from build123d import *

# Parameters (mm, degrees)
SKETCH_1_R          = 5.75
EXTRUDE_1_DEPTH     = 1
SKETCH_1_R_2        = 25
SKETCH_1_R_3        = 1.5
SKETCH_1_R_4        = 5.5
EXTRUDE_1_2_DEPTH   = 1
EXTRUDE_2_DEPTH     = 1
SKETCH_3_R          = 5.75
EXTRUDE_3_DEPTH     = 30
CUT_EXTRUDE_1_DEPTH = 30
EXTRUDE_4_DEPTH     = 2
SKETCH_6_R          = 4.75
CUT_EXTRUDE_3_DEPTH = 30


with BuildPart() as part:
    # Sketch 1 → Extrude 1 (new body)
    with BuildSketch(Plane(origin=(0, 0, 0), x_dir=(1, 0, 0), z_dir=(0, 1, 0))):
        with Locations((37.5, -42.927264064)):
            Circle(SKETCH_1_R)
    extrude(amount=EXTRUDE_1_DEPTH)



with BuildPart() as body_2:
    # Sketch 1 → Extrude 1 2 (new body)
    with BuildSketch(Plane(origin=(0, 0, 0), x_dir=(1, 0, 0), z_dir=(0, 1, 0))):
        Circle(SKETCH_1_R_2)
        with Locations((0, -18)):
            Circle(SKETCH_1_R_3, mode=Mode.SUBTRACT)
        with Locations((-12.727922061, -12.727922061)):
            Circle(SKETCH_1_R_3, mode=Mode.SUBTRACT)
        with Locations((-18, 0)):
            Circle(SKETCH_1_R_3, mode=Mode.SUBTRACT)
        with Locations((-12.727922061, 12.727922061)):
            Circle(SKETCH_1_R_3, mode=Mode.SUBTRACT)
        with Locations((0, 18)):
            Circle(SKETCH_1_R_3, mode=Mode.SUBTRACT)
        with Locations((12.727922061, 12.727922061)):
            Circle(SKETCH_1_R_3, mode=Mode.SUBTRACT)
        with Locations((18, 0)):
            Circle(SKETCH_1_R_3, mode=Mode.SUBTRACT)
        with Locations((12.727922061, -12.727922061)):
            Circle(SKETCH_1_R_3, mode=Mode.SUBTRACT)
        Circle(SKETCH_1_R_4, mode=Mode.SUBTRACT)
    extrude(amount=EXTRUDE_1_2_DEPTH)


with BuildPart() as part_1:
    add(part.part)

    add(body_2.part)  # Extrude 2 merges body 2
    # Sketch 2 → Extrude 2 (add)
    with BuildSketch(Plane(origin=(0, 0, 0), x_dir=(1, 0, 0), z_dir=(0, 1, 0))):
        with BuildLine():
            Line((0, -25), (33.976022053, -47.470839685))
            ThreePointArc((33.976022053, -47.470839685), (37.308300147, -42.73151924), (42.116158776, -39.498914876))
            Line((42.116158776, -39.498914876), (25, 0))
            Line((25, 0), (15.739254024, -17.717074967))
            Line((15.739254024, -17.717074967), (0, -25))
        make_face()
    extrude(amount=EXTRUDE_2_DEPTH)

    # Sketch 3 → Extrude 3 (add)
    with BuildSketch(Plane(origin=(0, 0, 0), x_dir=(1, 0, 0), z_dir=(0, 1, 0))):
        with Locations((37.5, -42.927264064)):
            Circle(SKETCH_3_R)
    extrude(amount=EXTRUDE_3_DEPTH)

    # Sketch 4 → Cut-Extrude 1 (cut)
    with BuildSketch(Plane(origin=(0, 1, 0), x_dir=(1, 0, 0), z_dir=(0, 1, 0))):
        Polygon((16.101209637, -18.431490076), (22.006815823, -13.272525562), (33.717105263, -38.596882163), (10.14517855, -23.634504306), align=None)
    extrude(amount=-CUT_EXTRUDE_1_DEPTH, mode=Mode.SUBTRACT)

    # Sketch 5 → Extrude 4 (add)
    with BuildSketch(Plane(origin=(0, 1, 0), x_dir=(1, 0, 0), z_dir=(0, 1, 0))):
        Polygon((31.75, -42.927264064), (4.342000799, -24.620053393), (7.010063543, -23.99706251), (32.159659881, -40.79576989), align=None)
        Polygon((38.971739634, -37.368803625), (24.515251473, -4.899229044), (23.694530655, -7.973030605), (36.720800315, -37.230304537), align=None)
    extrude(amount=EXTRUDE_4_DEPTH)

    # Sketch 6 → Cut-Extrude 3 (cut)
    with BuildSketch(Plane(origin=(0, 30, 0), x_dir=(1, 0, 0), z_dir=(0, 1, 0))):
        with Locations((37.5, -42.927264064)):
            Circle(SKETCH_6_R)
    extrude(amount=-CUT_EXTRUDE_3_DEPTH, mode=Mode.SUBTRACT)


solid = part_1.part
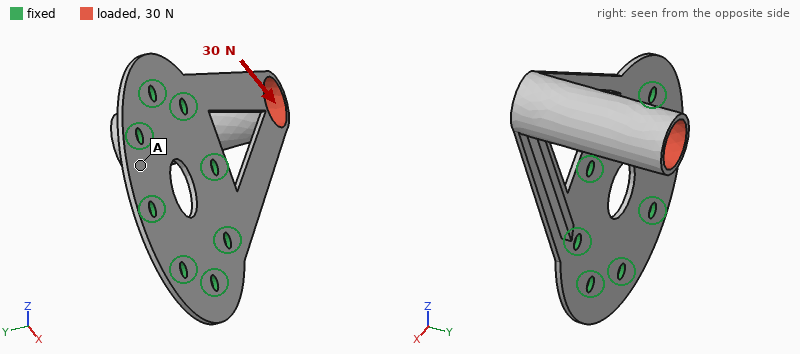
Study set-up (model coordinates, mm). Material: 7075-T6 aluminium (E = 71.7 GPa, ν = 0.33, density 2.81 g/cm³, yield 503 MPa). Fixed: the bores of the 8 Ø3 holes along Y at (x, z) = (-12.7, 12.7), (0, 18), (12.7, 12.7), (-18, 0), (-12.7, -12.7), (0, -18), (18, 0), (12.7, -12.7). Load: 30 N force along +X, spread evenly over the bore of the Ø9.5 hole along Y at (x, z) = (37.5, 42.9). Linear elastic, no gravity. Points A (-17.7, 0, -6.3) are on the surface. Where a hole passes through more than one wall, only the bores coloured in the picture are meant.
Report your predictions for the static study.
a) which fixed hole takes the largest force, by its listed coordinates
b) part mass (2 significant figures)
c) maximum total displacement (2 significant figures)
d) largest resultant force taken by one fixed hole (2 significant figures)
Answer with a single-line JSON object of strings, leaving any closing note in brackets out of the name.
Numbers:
{"which fixed hole takes the largest force, by its listed coordinates": "(0, 18)", "part mass": "10.0 g", "maximum total displacement": "1.1 mm", "largest resultant force taken by one fixed hole": "41 N"}
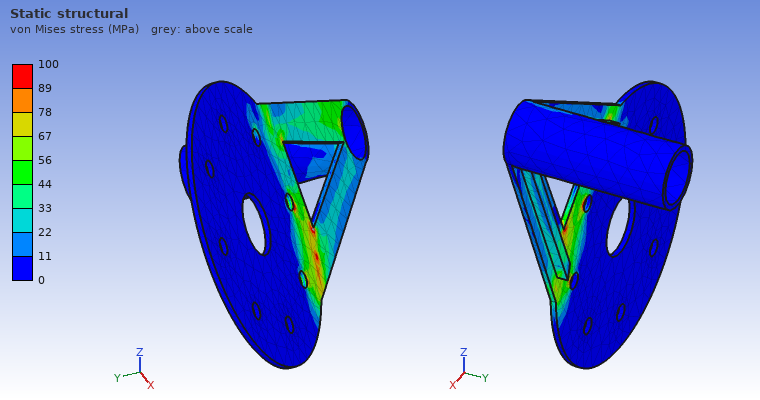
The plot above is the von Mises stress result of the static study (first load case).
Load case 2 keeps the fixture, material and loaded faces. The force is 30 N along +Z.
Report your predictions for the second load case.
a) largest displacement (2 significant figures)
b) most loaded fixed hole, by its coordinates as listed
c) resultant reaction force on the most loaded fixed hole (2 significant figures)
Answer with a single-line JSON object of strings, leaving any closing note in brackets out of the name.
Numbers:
{"largest displacement": "1.1 mm", "most loaded fixed hole, by its coordinates as listed": "(18, 0)", "resultant reaction force on the most loaded fixed hole": "39 N"}
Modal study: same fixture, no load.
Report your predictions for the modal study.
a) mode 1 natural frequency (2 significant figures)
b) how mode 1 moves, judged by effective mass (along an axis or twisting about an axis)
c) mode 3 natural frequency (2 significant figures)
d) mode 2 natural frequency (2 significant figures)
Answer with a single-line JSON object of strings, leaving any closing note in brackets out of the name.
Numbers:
{"mode 1 natural frequency": "310 Hz", "how mode 1 moves, judged by effective mass": "along Y", "mode 3 natural frequency": "1700 Hz", "mode 2 natural frequency": "730 Hz"}
